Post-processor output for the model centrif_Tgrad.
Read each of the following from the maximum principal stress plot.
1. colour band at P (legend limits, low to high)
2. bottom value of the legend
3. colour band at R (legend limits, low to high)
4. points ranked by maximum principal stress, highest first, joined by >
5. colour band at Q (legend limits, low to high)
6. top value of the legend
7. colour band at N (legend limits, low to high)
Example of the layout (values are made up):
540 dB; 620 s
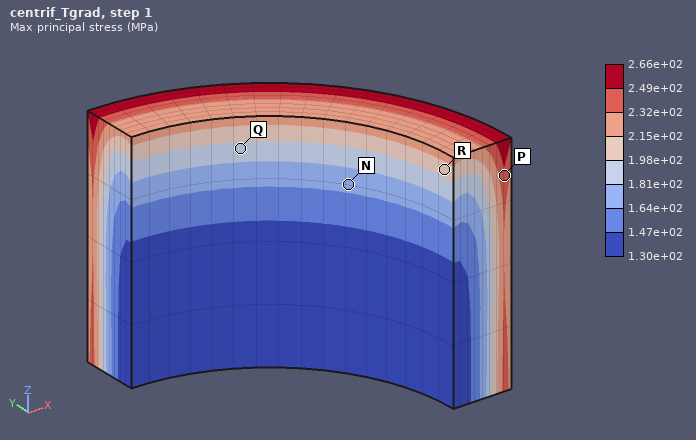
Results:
2.32e+02 to 2.49e+02 MPa; 1.30e+02 MPa; 1.98e+02 to 2.15e+02 MPa; P > R > Q > N; 1.81e+02 to 1.98e+02 MPa; 2.66e+02 MPa; 1.64e+02 to 1.81e+02 MPa
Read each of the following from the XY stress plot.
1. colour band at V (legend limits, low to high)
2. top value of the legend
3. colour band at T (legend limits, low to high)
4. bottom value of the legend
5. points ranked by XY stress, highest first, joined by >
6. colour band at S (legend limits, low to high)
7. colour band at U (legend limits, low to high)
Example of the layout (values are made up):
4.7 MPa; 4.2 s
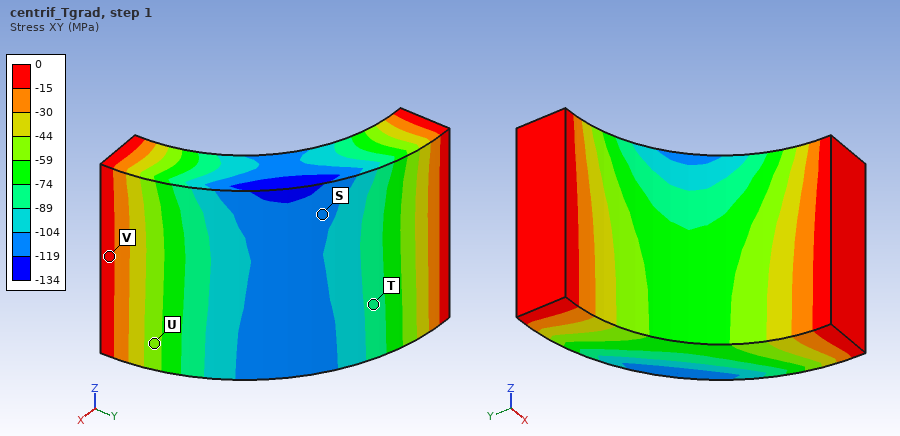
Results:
-15 to 0 MPa; 0 MPa; -89 to -74 MPa; -134 MPa; V > U > T > S; -119 to -104 MPa; -59 to -44 MPa
